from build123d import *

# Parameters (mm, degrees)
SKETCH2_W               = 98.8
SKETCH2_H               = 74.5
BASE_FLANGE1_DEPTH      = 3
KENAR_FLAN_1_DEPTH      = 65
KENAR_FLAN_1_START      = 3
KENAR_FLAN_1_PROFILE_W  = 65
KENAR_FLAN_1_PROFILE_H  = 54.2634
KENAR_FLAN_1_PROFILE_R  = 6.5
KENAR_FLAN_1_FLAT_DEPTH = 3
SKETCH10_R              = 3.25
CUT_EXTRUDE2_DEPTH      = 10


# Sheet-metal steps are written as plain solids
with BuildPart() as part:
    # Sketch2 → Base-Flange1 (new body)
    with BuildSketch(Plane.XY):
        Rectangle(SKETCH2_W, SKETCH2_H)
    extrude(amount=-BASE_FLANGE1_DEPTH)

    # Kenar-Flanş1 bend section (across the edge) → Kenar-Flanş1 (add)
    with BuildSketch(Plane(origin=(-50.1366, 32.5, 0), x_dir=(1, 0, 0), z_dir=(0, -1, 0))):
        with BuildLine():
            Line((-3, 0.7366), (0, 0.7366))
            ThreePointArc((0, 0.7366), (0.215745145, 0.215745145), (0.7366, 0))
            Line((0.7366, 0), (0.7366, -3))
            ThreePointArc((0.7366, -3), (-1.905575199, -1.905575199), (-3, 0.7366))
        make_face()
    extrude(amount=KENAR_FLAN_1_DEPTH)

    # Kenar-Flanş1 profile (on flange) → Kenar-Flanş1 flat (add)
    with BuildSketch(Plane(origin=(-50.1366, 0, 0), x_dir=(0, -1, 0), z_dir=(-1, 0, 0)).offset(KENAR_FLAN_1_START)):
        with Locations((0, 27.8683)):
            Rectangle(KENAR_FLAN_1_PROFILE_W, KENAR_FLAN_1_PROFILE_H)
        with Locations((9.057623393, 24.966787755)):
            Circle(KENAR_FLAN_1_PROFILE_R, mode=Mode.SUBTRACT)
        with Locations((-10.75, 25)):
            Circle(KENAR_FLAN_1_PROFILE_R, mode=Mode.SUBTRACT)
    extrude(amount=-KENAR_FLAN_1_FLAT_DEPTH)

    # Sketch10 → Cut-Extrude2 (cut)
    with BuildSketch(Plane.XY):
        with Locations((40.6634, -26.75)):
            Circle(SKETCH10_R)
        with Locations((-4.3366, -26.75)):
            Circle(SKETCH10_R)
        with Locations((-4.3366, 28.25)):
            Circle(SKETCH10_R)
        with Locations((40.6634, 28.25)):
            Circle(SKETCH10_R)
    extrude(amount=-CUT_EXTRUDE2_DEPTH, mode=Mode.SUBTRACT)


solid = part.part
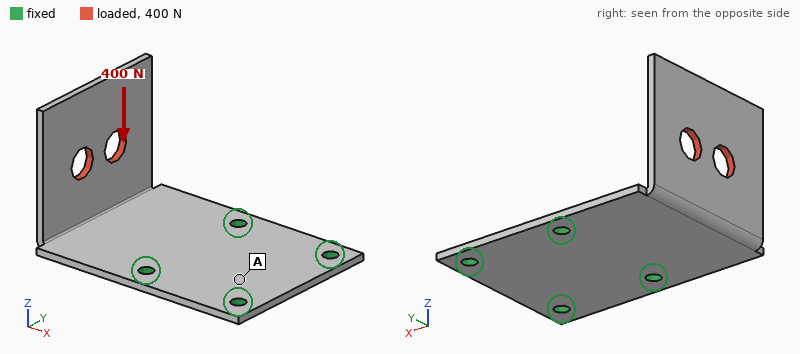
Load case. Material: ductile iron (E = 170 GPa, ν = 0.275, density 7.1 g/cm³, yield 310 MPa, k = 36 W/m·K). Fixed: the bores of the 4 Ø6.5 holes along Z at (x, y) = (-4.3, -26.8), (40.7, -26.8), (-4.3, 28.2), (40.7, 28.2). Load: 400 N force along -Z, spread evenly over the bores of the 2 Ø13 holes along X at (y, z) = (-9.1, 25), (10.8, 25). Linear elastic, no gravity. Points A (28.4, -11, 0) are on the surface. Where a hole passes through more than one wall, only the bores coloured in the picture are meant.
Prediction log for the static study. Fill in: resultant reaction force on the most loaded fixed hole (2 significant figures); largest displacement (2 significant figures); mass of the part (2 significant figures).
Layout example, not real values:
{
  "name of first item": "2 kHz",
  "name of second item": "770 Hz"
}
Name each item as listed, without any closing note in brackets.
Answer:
{
  "resultant reaction force on the most loaded fixed hole": "240 N",
  "largest displacement": "1.0 mm",
  "mass of the part": "230 g"
}
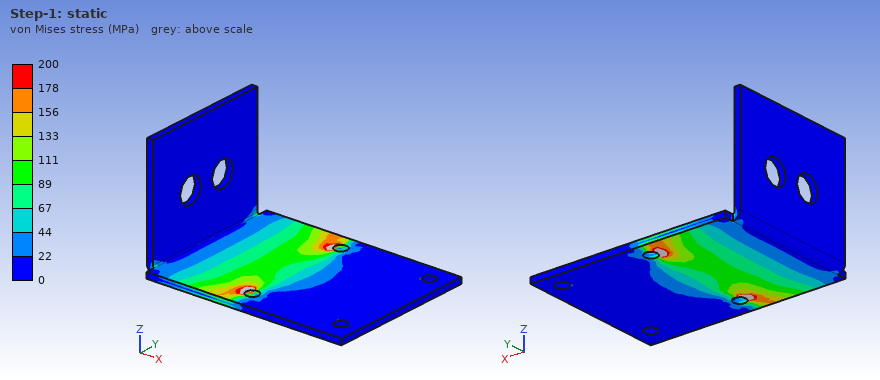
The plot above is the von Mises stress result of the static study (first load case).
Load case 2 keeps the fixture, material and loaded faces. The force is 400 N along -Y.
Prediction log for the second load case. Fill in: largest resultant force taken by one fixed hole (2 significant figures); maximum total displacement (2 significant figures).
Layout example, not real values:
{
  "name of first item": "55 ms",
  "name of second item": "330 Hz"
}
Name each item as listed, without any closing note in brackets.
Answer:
{
  "largest resultant force taken by one fixed hole": "410 N",
  "maximum total displacement": "0.38 mm"
}
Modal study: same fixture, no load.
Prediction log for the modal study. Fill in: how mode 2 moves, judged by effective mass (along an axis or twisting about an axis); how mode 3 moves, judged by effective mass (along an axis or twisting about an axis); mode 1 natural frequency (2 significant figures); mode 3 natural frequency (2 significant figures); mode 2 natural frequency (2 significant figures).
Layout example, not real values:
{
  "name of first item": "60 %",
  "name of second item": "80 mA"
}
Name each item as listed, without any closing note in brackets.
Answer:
{
  "how mode 2 moves, judged by effective mass": "along Y",
  "how mode 3 moves, judged by effective mass": "along Z",
  "mode 1 natural frequency": "320 Hz",
  "mode 3 natural frequency": "830 Hz",
  "mode 2 natural frequency": "630 Hz"
}
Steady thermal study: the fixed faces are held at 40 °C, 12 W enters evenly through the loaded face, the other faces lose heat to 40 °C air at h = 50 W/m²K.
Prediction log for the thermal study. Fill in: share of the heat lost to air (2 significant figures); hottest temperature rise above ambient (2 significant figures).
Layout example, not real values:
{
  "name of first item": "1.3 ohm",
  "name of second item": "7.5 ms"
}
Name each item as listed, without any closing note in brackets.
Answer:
{
  "share of the heat lost to air": "89 %",
  "hottest temperature rise above ambient": "40 K"
}
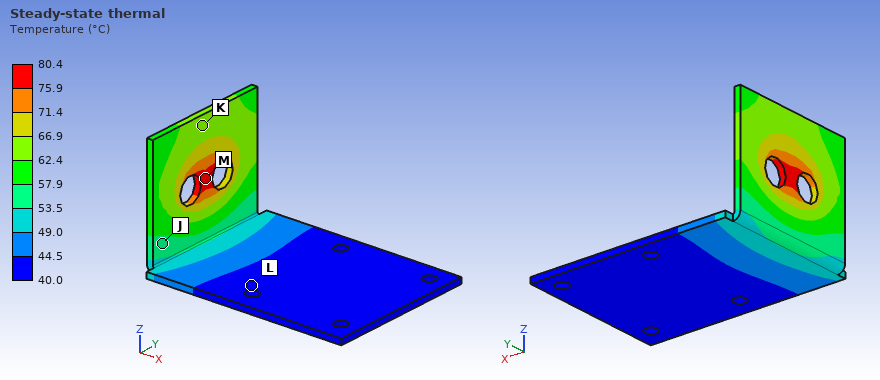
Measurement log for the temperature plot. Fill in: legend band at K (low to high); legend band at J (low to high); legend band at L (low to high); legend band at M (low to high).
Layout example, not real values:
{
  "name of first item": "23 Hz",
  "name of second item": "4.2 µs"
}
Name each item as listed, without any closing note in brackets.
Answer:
{
  "legend band at K": "62.4 to 66.9 °C",
  "legend band at J": "53.5 to 57.9 °C",
  "legend band at L": "40.0 to 44.5 °C",
  "legend band at M": "75.9 to 80.4 °C"
}
